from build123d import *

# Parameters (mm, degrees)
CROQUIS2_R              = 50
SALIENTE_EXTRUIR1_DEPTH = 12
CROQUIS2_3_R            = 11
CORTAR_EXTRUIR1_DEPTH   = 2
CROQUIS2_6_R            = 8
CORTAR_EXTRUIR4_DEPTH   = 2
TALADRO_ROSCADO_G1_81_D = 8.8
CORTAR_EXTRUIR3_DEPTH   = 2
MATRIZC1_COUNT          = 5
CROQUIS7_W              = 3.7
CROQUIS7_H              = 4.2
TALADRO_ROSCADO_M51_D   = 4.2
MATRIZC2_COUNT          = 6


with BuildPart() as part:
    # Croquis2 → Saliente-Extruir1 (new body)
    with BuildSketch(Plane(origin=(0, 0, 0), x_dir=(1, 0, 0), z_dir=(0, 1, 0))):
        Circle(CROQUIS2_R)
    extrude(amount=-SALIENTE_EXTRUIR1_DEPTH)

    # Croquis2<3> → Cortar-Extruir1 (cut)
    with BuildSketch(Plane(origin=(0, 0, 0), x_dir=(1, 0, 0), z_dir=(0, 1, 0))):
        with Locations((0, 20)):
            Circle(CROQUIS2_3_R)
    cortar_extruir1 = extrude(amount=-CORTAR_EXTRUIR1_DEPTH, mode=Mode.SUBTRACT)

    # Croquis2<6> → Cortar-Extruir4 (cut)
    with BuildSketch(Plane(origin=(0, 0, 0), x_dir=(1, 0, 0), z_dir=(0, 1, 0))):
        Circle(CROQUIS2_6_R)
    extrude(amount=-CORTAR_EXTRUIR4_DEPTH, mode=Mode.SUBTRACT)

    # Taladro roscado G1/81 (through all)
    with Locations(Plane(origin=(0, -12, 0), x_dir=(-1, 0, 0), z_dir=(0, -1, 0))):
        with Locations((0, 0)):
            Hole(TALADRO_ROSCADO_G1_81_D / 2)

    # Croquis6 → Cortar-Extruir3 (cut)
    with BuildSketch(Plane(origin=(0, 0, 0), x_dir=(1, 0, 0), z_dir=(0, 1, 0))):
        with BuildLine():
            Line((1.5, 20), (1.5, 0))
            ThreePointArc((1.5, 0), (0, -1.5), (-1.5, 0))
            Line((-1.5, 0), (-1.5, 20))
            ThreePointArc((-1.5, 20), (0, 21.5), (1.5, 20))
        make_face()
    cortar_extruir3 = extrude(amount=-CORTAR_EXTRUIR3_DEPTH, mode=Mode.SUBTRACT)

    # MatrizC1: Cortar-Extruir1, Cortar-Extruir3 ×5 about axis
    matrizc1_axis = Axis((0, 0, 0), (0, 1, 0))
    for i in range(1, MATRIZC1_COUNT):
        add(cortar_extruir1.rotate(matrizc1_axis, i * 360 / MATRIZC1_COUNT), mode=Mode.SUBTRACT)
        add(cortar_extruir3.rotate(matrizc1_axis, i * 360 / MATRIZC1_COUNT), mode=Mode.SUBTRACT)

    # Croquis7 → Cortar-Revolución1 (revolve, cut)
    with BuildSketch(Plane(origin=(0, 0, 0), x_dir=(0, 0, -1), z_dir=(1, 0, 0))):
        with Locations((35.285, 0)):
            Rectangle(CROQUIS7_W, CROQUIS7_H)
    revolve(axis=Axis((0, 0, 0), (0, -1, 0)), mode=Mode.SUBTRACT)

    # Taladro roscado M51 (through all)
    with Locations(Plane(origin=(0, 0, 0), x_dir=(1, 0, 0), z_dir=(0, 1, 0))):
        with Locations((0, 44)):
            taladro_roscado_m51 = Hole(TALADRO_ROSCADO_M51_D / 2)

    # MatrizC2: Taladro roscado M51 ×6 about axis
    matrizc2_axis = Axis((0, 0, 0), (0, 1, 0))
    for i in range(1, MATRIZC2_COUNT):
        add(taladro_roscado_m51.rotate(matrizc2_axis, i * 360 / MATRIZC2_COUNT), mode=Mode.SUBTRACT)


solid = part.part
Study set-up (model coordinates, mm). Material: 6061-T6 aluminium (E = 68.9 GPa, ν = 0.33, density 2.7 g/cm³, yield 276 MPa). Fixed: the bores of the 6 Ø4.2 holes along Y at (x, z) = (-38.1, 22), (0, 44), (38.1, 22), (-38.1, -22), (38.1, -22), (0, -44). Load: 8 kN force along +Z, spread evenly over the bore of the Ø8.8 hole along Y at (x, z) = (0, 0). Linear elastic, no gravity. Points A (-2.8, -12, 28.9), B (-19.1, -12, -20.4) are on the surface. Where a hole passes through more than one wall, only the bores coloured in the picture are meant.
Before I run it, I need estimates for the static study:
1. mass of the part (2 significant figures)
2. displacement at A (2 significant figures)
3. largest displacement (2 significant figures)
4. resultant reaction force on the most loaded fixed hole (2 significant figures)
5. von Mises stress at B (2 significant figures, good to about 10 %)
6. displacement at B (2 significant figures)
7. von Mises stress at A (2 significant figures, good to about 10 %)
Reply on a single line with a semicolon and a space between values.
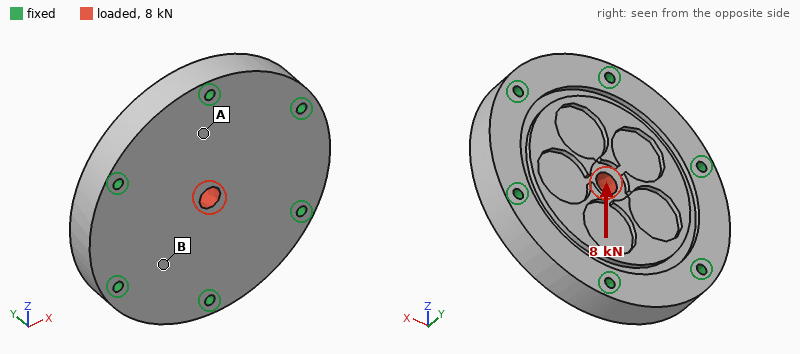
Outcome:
230 g; 2.7 µm; 8.4 µm; 2.0 kN; 4.4 MPa; 2.7 µm; 11 MPa
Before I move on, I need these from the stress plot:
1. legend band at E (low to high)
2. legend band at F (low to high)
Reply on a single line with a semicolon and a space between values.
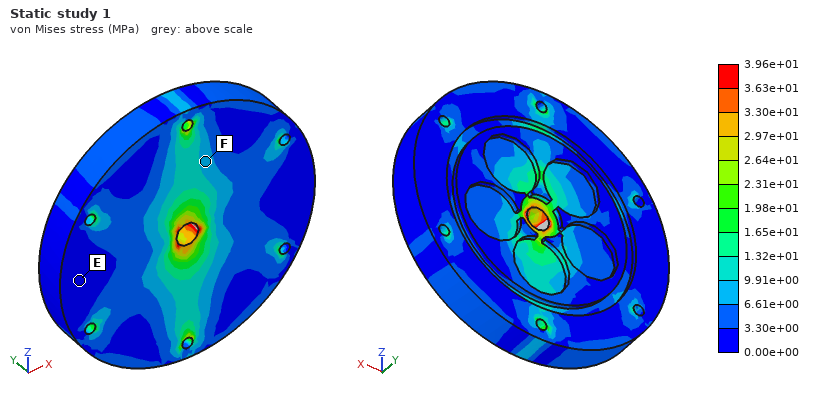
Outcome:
0.00e+00 to 3.30e+00 MPa; 6.61e+00 to 9.91e+00 MPa
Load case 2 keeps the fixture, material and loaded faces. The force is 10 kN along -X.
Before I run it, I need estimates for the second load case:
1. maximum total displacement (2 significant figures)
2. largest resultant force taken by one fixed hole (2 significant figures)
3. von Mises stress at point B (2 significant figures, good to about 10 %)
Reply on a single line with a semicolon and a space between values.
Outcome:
11 µm; 2.2 kN; 8.4 MPa
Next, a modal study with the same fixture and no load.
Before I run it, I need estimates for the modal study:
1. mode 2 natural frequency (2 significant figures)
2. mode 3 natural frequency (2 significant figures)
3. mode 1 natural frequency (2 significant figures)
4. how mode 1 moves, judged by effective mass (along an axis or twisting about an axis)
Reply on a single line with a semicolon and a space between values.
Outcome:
18 kHz; 18 kHz; 9600 Hz; along Y
